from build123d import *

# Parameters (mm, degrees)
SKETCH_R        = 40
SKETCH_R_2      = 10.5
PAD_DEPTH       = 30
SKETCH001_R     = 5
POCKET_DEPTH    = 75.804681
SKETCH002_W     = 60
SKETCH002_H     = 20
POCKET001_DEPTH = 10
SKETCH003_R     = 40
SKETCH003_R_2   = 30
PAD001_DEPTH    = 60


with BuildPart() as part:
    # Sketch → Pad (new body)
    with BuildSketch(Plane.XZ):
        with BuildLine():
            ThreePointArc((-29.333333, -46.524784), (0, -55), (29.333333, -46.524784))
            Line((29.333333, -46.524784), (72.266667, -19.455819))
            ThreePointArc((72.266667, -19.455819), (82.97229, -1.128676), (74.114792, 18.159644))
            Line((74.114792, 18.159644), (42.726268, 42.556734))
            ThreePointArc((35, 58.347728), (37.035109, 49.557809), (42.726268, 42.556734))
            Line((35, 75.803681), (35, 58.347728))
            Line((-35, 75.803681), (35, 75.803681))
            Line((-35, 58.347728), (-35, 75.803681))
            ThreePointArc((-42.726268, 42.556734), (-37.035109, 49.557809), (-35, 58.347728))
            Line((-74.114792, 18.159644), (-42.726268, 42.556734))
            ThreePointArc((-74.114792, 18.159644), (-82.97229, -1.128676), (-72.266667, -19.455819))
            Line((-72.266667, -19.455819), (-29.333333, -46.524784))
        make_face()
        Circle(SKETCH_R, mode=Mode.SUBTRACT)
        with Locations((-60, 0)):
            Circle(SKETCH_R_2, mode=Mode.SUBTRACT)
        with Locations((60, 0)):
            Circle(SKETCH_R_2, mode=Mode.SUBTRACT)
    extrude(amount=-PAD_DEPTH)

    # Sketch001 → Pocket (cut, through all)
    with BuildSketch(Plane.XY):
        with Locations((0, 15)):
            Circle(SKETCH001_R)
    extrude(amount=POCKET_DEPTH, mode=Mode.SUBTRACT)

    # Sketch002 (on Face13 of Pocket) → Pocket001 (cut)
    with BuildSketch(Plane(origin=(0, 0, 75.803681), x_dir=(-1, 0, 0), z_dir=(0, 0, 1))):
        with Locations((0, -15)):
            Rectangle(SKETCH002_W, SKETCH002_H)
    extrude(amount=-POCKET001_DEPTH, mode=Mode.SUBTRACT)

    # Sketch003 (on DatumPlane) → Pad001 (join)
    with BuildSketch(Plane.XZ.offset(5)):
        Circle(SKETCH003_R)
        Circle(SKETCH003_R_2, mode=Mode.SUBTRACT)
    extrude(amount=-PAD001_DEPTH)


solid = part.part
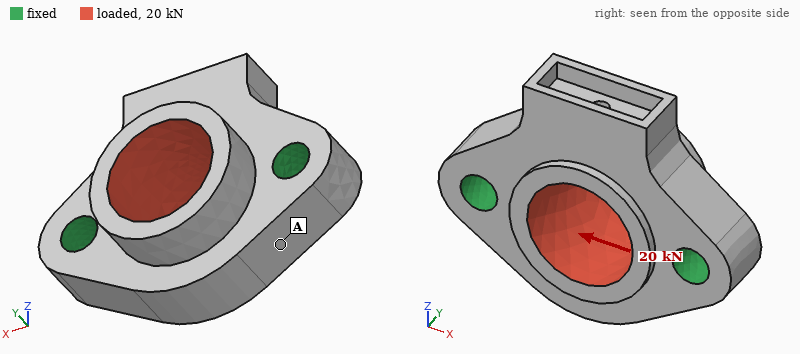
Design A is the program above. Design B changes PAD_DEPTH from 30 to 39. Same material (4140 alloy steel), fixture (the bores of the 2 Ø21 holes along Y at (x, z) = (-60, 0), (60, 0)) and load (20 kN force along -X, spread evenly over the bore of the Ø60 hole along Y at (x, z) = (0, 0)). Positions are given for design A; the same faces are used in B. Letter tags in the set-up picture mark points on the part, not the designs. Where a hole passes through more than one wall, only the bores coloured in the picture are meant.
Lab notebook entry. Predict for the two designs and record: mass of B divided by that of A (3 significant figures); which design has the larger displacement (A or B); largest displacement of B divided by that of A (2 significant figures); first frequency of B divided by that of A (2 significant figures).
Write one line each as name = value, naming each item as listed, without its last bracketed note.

mass of B divided by that of A = 1.21
which design has the larger displacement = A
largest displacement of B divided by that of A = 0.61
first frequency of B divided by that of A = 1.2
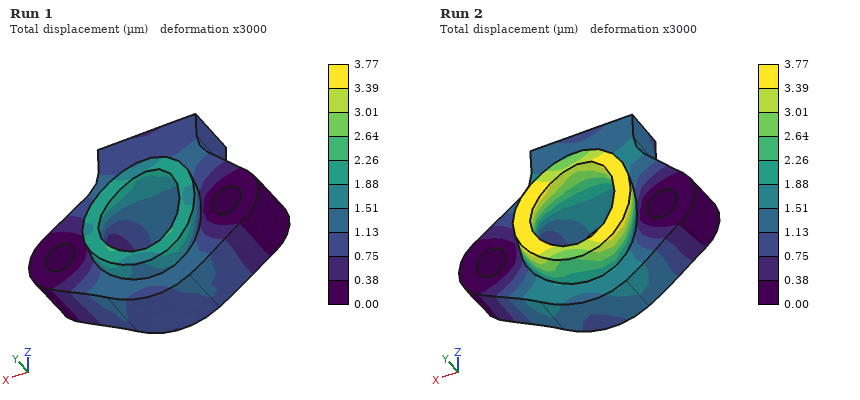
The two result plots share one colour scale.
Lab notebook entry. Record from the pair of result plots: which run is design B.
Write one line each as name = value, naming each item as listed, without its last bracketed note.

which run is design B = Run 1
